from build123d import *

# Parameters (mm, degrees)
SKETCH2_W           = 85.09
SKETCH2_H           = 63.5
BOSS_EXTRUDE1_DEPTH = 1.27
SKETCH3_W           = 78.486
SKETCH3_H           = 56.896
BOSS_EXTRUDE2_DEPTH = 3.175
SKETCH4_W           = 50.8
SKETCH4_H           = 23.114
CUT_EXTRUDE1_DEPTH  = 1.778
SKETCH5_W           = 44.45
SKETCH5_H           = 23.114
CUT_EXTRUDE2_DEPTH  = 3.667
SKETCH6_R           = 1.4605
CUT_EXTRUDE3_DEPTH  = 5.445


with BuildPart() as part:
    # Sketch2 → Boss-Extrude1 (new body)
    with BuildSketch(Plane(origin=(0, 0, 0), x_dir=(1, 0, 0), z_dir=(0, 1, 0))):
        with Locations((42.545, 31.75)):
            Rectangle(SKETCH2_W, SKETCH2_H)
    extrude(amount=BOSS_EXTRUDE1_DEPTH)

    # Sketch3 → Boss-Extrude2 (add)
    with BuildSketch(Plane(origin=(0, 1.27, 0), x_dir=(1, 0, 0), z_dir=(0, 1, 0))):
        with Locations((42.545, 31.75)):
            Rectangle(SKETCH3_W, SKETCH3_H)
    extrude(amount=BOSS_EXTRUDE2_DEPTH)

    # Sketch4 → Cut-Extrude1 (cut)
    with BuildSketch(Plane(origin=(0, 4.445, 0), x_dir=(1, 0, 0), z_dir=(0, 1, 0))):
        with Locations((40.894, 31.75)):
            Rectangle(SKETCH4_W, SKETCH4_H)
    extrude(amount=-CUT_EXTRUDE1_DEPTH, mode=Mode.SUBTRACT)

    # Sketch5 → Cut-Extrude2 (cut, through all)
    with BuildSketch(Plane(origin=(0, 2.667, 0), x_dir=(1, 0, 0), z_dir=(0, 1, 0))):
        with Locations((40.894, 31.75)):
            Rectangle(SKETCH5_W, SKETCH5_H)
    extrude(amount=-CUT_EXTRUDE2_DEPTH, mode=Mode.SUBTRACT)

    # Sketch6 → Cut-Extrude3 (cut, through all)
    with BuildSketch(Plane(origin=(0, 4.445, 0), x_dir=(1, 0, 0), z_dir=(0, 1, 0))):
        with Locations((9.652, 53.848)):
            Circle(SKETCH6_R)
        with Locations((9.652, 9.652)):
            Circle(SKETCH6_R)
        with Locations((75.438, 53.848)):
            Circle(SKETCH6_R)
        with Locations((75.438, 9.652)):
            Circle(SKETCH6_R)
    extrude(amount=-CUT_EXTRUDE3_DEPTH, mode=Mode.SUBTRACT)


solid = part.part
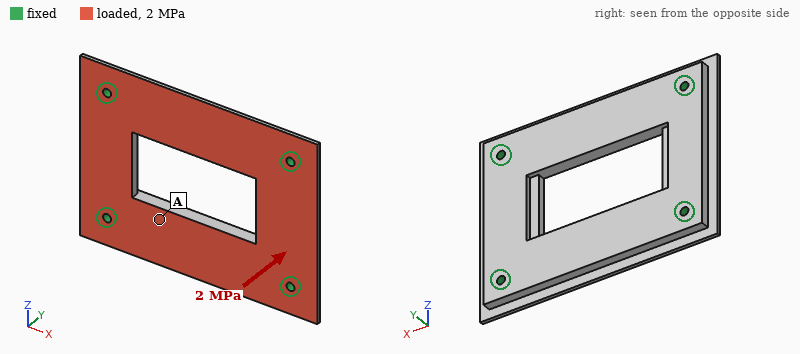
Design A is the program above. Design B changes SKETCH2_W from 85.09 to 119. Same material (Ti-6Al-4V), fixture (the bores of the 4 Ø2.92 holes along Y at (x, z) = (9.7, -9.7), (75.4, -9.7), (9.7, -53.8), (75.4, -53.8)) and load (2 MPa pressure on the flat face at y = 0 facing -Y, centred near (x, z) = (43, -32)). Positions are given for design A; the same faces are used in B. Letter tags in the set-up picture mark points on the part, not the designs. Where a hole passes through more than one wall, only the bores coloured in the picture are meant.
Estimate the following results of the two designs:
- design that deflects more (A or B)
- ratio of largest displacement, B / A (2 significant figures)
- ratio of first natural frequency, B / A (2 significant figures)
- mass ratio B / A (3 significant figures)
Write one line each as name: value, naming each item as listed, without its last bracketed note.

design that deflects more: B
ratio of largest displacement, B / A: 14
ratio of first natural frequency, B / A: 0.49
mass ratio B / A: 1.17
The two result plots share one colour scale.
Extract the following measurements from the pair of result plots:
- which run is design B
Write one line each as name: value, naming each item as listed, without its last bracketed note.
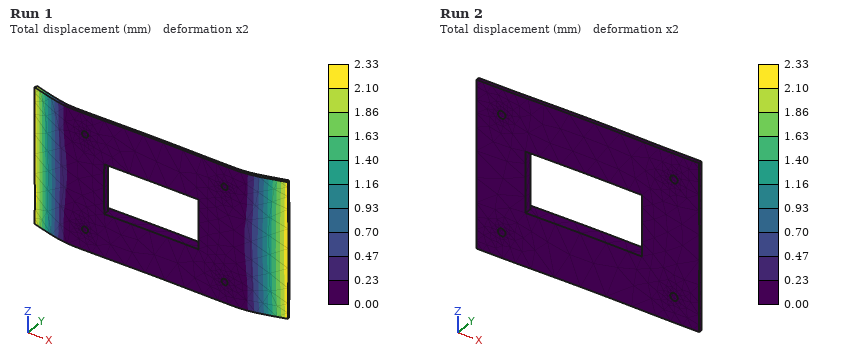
which run is design B: Run 1
